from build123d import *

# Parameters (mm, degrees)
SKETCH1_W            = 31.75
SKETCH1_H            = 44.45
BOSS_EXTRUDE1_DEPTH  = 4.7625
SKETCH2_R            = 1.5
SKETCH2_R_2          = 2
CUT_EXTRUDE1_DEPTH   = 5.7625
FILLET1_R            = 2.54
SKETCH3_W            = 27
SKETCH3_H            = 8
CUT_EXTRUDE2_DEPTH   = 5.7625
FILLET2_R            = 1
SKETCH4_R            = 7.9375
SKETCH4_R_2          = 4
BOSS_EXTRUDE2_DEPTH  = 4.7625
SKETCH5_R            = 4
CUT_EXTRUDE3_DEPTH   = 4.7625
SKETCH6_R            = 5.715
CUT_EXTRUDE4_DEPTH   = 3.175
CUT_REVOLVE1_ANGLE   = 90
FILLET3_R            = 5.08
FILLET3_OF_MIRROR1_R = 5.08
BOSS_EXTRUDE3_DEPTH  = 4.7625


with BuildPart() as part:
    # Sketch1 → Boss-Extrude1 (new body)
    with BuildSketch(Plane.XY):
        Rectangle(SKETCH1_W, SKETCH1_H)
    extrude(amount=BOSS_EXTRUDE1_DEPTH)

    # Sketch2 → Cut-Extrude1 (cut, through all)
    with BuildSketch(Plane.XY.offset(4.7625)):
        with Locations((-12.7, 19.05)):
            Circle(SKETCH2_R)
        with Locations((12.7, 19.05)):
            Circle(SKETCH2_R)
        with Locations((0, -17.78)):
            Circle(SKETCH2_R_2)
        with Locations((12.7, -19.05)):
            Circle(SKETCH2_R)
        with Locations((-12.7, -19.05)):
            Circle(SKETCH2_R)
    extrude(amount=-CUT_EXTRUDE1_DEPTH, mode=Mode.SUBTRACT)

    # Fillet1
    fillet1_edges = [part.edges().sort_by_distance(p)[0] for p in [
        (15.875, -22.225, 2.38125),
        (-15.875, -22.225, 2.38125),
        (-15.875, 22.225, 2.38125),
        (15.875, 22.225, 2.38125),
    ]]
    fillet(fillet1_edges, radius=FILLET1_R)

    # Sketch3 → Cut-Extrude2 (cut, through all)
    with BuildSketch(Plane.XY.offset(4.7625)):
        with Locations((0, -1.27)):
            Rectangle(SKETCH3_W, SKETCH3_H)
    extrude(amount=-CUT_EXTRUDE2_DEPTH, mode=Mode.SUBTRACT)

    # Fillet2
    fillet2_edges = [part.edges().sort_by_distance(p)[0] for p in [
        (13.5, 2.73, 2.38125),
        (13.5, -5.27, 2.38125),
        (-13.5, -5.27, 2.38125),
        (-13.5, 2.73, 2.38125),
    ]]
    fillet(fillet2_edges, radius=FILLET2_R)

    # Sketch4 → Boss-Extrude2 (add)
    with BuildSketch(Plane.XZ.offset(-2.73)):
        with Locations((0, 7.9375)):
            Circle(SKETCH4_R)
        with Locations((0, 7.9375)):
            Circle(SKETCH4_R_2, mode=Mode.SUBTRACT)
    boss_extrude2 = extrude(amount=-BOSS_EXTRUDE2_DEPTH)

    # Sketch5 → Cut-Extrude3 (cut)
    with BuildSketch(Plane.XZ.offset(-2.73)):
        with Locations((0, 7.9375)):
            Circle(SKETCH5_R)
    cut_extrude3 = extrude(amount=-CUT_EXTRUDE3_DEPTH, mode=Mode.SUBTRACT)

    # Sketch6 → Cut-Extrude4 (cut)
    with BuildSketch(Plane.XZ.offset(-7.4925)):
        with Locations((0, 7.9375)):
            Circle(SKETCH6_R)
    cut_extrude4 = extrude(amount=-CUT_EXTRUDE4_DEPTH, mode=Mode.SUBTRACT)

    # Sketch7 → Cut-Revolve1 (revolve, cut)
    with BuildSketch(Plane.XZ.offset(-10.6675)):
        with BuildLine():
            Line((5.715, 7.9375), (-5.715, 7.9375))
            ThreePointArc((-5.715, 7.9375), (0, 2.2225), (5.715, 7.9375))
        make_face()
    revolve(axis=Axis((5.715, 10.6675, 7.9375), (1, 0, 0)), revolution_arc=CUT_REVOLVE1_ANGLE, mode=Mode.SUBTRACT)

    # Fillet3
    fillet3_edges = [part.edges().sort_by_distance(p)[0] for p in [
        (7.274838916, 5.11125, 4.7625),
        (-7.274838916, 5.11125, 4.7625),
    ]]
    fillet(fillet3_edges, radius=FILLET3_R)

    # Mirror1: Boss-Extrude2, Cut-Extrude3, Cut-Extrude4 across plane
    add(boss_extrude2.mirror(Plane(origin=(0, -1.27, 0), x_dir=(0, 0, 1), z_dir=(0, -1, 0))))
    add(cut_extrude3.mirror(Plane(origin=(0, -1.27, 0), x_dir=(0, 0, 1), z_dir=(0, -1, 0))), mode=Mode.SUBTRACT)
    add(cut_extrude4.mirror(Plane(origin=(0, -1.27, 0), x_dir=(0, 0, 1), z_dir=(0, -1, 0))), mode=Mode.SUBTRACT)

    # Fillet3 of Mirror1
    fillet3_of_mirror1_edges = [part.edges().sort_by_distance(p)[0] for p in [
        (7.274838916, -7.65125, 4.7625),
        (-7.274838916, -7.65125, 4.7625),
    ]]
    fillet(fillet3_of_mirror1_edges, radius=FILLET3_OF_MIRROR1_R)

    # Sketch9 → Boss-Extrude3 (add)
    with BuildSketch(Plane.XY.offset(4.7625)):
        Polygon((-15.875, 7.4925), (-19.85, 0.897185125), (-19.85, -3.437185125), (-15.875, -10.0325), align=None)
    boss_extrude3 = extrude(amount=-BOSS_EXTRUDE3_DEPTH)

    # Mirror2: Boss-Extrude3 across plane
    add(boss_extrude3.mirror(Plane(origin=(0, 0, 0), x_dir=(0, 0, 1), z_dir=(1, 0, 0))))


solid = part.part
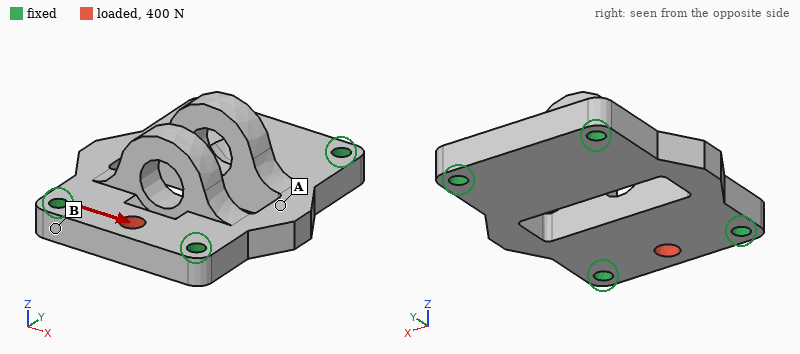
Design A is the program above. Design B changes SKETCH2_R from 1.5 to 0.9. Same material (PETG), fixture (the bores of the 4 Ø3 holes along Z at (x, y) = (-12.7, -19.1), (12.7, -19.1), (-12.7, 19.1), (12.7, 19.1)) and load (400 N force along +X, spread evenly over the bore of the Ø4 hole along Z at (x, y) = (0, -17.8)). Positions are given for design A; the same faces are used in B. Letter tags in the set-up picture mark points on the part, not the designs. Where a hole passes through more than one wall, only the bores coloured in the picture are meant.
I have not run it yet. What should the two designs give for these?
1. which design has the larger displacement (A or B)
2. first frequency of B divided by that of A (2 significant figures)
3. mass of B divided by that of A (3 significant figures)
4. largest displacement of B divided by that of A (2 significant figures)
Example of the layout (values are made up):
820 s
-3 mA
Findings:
B
0.90
1.01
1.1
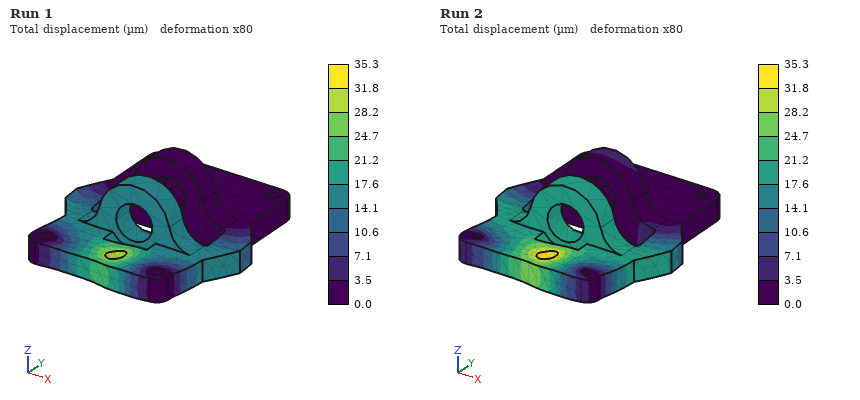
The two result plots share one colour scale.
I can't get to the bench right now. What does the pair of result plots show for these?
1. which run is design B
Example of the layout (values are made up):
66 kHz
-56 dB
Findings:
Run 2
